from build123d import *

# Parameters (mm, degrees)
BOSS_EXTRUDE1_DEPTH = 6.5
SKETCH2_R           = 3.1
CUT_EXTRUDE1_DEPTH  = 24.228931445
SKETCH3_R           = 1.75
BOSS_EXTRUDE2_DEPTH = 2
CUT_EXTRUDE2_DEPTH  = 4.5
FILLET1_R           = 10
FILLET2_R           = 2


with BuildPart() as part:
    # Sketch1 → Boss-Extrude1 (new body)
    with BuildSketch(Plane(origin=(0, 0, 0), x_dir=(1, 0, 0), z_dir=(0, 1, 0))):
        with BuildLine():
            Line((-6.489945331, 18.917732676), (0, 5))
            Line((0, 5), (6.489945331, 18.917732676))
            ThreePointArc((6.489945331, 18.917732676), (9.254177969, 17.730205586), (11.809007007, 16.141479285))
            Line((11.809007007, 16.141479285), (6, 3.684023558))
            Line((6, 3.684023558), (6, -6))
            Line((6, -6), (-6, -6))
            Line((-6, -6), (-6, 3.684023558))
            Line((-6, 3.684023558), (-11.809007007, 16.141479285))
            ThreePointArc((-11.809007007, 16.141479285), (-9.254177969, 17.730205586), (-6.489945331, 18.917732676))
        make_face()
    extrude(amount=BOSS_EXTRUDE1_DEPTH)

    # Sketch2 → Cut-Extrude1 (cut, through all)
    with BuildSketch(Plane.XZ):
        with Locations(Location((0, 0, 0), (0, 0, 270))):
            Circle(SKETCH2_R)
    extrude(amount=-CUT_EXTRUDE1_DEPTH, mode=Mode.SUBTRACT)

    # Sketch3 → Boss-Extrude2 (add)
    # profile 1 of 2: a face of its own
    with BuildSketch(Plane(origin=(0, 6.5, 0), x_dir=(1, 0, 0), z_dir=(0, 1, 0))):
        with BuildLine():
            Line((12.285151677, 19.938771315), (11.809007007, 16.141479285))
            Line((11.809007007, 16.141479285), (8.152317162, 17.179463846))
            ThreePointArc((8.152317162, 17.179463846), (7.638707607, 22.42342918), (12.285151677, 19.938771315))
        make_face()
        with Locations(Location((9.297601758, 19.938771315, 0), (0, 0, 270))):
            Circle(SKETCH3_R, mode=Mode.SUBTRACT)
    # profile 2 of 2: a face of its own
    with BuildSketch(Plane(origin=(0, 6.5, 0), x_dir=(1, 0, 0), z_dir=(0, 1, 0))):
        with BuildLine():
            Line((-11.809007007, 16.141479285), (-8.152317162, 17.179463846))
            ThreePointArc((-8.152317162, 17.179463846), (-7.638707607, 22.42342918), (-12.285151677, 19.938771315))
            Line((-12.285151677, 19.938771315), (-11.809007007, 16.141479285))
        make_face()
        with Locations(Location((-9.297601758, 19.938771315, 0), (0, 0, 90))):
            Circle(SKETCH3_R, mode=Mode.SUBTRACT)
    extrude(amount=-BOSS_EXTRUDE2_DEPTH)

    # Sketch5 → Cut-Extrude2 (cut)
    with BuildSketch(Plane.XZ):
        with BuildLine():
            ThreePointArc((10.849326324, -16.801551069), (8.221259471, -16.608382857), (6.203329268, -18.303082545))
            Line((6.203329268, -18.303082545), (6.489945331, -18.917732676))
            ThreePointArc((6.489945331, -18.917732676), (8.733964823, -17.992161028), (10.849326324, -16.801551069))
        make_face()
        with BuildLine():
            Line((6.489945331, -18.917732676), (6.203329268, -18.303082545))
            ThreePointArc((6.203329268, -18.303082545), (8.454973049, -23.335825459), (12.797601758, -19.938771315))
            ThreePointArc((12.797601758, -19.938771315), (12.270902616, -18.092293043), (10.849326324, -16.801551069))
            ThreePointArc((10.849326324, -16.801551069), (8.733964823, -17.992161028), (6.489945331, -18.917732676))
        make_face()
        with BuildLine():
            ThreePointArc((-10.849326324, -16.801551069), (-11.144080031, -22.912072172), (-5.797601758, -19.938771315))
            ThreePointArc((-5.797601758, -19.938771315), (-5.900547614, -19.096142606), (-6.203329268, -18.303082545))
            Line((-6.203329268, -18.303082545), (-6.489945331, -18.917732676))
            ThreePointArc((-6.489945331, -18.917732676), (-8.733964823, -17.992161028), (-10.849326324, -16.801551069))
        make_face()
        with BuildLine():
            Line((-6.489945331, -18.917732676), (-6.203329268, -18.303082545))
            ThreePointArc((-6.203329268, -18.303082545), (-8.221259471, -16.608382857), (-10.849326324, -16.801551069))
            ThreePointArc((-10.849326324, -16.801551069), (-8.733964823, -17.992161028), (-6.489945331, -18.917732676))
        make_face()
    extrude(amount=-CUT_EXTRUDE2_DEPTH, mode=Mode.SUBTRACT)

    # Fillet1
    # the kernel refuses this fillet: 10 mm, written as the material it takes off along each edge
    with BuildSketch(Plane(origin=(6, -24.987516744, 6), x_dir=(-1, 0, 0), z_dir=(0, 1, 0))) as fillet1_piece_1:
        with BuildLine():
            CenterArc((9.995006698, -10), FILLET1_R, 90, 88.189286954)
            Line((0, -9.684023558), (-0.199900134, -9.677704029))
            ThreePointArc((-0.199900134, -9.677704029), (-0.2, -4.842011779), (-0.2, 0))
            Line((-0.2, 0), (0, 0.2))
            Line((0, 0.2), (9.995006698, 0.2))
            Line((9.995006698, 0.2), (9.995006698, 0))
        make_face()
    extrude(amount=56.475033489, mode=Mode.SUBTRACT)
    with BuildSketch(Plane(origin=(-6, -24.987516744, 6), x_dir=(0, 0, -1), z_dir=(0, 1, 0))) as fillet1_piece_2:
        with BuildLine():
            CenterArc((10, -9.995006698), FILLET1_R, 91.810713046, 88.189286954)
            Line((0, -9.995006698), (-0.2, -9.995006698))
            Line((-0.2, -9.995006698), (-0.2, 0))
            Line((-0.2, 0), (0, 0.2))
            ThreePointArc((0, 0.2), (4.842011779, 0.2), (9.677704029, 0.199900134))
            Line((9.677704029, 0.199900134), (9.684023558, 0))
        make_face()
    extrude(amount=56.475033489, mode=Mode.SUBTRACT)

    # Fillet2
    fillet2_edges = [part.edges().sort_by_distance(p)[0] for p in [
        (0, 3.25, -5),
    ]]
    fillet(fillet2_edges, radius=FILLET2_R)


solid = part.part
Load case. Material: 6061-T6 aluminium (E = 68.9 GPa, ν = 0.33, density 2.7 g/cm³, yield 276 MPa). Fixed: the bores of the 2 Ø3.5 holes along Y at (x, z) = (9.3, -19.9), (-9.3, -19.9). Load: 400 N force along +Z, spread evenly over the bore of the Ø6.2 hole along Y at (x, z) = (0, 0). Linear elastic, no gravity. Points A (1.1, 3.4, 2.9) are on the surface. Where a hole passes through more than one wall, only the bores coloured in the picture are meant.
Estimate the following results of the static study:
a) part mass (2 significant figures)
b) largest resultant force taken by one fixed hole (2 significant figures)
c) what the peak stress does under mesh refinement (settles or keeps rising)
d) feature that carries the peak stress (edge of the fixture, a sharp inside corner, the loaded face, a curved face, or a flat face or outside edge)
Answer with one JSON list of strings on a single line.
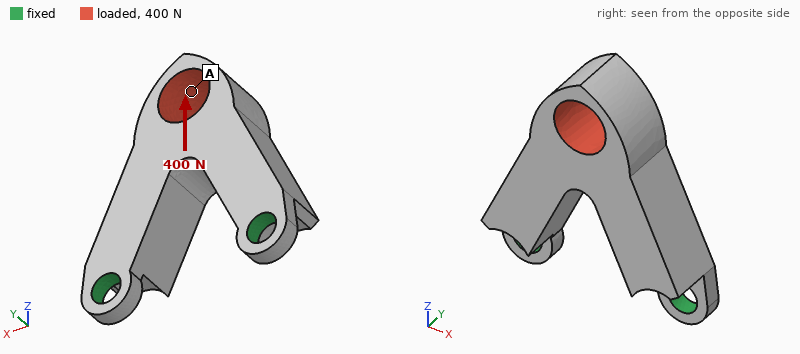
["4.2 g", "210 N", "keeps rising", "a sharp inside corner"]
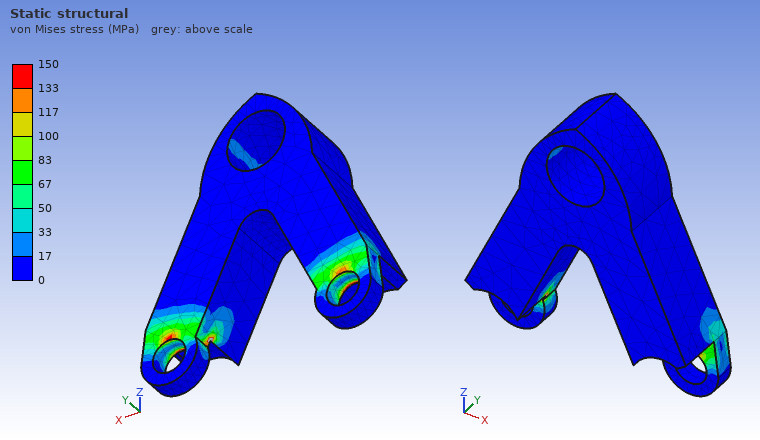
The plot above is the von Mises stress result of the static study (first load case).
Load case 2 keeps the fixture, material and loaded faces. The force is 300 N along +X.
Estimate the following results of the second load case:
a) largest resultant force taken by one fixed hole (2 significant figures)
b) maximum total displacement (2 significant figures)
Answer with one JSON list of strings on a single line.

["320 N", "16 µm"]
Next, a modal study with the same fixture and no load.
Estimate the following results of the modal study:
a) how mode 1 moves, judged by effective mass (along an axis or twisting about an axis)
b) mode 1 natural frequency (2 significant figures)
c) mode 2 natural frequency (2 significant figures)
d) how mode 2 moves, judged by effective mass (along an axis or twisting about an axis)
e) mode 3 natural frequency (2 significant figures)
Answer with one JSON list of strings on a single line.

["along Y", "3200 Hz", "19 kHz", "along X", "21 kHz"]
